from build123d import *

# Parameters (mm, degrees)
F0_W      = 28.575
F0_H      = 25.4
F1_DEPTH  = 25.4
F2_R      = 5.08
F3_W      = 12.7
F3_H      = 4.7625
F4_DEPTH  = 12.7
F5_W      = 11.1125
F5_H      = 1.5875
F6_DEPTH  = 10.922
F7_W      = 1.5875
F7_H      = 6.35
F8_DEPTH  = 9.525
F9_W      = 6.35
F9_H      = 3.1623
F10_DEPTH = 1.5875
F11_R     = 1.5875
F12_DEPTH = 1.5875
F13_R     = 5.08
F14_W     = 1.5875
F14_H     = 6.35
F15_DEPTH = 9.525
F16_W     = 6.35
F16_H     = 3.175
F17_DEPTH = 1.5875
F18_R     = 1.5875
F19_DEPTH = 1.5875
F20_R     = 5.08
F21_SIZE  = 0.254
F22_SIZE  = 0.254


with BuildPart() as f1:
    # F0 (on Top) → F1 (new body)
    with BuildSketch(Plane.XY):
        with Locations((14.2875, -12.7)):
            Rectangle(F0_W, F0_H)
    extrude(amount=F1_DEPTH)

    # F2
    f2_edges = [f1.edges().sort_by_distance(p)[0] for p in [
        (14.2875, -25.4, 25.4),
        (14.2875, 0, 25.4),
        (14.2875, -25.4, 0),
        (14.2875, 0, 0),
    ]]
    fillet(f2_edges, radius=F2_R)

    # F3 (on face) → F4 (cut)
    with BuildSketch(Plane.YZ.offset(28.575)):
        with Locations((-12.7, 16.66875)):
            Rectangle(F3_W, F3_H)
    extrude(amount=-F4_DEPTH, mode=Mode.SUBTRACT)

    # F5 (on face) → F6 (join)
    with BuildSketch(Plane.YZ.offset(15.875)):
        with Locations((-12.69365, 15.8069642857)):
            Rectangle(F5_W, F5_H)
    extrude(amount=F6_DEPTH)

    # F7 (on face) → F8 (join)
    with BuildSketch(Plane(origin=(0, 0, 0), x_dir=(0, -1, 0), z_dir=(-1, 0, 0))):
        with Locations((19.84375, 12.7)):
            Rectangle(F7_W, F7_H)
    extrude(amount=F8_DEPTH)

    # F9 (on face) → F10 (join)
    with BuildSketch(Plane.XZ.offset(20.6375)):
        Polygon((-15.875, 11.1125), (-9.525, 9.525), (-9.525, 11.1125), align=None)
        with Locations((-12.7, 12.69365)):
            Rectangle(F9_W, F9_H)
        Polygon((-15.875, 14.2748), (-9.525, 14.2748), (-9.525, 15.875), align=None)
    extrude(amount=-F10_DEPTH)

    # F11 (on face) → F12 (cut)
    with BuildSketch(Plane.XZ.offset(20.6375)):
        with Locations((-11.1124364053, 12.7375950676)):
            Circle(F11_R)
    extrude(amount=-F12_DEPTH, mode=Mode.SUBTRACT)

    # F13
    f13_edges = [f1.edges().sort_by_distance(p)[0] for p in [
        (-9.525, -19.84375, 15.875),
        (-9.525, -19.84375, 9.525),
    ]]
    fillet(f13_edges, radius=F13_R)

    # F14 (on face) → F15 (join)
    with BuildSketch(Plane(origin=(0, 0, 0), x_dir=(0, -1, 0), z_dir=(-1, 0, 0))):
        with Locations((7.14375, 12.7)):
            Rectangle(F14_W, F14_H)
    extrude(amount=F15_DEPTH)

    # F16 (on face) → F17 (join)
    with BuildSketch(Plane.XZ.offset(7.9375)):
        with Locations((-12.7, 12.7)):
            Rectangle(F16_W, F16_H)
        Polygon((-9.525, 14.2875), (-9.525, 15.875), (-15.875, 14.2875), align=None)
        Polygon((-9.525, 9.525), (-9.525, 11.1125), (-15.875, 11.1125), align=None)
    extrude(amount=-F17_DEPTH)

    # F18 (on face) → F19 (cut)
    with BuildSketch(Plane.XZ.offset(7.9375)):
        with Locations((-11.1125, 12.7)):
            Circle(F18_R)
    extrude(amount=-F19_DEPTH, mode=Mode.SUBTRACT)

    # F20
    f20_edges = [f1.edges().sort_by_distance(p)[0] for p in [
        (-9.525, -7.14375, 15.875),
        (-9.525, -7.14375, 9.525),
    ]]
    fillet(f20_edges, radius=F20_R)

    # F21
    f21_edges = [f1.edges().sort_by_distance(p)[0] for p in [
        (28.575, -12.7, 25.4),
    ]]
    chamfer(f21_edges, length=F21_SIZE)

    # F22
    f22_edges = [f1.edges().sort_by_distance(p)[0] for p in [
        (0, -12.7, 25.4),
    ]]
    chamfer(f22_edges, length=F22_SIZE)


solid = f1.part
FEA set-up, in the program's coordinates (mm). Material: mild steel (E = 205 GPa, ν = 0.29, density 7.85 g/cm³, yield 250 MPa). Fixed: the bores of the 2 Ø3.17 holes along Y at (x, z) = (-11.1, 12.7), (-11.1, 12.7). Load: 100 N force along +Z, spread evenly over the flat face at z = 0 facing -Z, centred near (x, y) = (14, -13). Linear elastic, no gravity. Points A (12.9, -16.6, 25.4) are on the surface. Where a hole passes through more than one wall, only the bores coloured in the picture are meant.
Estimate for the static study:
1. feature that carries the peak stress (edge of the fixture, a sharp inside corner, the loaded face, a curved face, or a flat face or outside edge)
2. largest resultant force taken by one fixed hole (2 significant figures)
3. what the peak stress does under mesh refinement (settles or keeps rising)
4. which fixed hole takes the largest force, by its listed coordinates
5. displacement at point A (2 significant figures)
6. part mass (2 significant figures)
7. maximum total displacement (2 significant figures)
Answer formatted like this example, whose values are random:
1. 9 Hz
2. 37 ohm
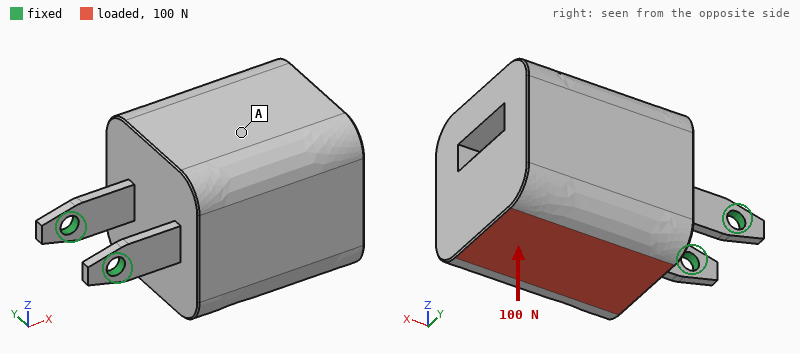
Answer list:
1. edge of the fixture
2. 56 N
3. keeps rising
4. (-11.1, 12.7)
5. 42 µm
6. 140 g
7. 68 µm
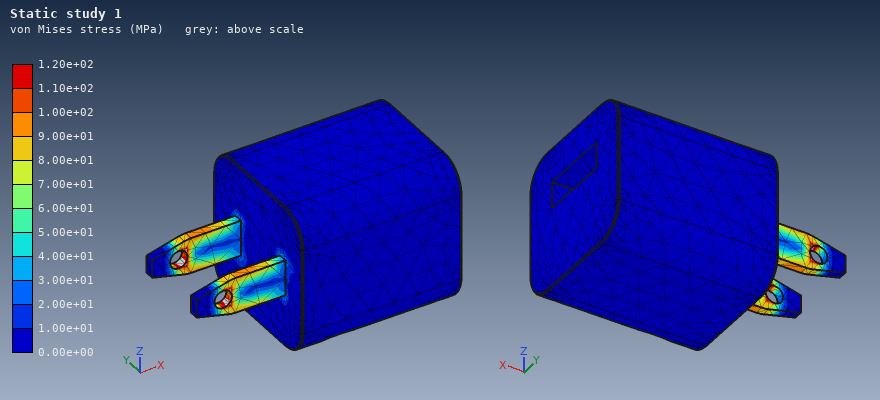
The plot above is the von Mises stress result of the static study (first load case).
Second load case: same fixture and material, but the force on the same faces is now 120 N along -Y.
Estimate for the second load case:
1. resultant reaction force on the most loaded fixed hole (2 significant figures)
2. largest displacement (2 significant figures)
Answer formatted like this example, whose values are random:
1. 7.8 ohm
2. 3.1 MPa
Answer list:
1. 220 N
2. 28 µm
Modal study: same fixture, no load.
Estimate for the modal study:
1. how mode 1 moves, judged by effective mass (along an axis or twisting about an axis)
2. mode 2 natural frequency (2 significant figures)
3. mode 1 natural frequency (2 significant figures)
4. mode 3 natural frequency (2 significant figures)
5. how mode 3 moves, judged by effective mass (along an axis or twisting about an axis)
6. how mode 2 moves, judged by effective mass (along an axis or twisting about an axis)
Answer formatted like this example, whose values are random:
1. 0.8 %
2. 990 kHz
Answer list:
1. along Z
2. 1200 Hz
3. 630 Hz
4. 2000 Hz
5. twisting about X
6. along Y
